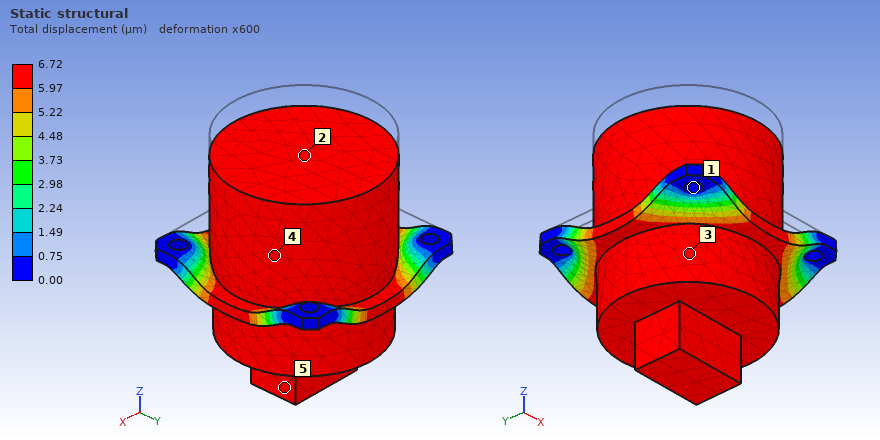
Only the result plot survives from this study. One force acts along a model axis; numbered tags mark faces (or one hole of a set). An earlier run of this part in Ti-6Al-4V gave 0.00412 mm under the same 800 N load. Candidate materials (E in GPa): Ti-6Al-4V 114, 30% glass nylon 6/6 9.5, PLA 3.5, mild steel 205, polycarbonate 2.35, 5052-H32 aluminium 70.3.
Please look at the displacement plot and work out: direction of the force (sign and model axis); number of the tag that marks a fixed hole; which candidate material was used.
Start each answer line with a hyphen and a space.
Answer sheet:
- -Z
- 1
- 5052-H32 aluminium
